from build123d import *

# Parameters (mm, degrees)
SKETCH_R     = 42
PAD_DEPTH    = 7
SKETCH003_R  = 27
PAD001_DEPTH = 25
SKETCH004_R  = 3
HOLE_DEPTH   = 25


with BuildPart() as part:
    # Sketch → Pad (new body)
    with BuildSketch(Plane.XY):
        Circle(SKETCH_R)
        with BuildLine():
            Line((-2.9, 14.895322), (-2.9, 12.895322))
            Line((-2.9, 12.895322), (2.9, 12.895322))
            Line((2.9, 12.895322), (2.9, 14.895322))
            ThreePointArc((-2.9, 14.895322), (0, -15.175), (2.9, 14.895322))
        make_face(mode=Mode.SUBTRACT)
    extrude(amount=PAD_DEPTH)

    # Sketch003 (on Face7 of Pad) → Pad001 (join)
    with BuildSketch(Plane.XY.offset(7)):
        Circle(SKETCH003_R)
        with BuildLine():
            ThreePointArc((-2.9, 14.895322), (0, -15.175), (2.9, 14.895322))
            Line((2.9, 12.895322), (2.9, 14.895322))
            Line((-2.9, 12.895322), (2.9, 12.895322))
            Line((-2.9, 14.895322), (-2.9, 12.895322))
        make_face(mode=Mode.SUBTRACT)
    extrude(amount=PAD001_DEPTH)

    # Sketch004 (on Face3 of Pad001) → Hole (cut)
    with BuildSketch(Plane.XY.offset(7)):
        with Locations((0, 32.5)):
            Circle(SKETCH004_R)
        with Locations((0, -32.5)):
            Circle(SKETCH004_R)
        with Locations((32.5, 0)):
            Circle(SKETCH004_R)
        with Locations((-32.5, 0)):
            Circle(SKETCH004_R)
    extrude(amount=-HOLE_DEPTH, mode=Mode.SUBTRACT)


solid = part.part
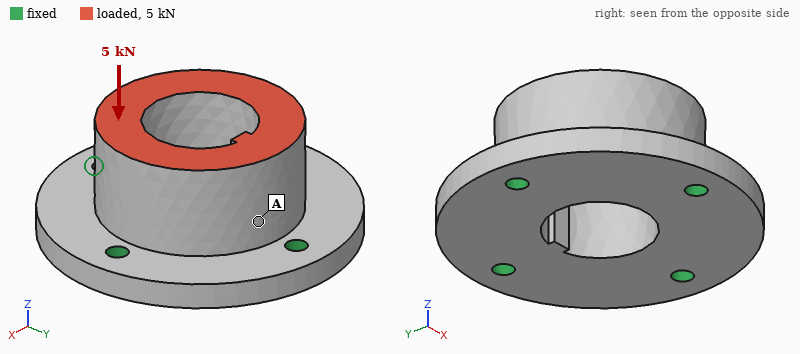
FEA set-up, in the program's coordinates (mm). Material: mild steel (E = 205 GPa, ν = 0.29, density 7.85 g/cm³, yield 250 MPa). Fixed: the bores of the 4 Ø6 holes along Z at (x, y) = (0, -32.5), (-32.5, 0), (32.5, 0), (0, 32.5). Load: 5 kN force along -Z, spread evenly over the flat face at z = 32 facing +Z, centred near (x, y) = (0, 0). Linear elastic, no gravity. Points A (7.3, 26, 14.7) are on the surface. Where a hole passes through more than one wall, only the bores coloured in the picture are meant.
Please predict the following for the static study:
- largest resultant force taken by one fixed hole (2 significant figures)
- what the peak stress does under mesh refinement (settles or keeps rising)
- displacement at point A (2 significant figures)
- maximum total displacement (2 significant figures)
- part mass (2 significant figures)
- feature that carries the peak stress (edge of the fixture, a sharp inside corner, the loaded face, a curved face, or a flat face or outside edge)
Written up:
1.3 kN
keeps rising
1.7 µm
2.0 µm
570 g
edge of the fixture
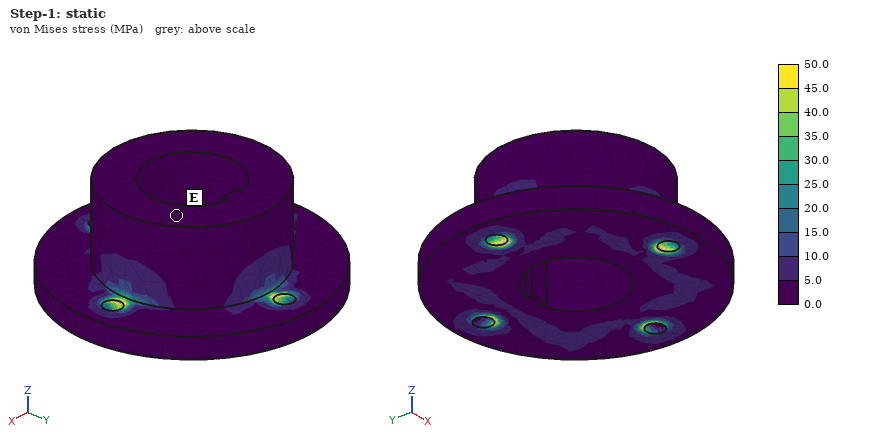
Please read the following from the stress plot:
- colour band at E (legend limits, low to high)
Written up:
0.0 to 5.0 MPa
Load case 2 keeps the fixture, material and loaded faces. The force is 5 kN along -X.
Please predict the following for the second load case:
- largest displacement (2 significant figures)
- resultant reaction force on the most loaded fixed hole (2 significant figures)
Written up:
6.6 µm
2.8 kN
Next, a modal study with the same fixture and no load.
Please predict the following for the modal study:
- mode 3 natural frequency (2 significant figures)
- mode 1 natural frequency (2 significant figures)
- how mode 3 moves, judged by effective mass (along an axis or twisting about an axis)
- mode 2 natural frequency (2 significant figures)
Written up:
13 kHz
11 kHz
along Z
11 kHz
